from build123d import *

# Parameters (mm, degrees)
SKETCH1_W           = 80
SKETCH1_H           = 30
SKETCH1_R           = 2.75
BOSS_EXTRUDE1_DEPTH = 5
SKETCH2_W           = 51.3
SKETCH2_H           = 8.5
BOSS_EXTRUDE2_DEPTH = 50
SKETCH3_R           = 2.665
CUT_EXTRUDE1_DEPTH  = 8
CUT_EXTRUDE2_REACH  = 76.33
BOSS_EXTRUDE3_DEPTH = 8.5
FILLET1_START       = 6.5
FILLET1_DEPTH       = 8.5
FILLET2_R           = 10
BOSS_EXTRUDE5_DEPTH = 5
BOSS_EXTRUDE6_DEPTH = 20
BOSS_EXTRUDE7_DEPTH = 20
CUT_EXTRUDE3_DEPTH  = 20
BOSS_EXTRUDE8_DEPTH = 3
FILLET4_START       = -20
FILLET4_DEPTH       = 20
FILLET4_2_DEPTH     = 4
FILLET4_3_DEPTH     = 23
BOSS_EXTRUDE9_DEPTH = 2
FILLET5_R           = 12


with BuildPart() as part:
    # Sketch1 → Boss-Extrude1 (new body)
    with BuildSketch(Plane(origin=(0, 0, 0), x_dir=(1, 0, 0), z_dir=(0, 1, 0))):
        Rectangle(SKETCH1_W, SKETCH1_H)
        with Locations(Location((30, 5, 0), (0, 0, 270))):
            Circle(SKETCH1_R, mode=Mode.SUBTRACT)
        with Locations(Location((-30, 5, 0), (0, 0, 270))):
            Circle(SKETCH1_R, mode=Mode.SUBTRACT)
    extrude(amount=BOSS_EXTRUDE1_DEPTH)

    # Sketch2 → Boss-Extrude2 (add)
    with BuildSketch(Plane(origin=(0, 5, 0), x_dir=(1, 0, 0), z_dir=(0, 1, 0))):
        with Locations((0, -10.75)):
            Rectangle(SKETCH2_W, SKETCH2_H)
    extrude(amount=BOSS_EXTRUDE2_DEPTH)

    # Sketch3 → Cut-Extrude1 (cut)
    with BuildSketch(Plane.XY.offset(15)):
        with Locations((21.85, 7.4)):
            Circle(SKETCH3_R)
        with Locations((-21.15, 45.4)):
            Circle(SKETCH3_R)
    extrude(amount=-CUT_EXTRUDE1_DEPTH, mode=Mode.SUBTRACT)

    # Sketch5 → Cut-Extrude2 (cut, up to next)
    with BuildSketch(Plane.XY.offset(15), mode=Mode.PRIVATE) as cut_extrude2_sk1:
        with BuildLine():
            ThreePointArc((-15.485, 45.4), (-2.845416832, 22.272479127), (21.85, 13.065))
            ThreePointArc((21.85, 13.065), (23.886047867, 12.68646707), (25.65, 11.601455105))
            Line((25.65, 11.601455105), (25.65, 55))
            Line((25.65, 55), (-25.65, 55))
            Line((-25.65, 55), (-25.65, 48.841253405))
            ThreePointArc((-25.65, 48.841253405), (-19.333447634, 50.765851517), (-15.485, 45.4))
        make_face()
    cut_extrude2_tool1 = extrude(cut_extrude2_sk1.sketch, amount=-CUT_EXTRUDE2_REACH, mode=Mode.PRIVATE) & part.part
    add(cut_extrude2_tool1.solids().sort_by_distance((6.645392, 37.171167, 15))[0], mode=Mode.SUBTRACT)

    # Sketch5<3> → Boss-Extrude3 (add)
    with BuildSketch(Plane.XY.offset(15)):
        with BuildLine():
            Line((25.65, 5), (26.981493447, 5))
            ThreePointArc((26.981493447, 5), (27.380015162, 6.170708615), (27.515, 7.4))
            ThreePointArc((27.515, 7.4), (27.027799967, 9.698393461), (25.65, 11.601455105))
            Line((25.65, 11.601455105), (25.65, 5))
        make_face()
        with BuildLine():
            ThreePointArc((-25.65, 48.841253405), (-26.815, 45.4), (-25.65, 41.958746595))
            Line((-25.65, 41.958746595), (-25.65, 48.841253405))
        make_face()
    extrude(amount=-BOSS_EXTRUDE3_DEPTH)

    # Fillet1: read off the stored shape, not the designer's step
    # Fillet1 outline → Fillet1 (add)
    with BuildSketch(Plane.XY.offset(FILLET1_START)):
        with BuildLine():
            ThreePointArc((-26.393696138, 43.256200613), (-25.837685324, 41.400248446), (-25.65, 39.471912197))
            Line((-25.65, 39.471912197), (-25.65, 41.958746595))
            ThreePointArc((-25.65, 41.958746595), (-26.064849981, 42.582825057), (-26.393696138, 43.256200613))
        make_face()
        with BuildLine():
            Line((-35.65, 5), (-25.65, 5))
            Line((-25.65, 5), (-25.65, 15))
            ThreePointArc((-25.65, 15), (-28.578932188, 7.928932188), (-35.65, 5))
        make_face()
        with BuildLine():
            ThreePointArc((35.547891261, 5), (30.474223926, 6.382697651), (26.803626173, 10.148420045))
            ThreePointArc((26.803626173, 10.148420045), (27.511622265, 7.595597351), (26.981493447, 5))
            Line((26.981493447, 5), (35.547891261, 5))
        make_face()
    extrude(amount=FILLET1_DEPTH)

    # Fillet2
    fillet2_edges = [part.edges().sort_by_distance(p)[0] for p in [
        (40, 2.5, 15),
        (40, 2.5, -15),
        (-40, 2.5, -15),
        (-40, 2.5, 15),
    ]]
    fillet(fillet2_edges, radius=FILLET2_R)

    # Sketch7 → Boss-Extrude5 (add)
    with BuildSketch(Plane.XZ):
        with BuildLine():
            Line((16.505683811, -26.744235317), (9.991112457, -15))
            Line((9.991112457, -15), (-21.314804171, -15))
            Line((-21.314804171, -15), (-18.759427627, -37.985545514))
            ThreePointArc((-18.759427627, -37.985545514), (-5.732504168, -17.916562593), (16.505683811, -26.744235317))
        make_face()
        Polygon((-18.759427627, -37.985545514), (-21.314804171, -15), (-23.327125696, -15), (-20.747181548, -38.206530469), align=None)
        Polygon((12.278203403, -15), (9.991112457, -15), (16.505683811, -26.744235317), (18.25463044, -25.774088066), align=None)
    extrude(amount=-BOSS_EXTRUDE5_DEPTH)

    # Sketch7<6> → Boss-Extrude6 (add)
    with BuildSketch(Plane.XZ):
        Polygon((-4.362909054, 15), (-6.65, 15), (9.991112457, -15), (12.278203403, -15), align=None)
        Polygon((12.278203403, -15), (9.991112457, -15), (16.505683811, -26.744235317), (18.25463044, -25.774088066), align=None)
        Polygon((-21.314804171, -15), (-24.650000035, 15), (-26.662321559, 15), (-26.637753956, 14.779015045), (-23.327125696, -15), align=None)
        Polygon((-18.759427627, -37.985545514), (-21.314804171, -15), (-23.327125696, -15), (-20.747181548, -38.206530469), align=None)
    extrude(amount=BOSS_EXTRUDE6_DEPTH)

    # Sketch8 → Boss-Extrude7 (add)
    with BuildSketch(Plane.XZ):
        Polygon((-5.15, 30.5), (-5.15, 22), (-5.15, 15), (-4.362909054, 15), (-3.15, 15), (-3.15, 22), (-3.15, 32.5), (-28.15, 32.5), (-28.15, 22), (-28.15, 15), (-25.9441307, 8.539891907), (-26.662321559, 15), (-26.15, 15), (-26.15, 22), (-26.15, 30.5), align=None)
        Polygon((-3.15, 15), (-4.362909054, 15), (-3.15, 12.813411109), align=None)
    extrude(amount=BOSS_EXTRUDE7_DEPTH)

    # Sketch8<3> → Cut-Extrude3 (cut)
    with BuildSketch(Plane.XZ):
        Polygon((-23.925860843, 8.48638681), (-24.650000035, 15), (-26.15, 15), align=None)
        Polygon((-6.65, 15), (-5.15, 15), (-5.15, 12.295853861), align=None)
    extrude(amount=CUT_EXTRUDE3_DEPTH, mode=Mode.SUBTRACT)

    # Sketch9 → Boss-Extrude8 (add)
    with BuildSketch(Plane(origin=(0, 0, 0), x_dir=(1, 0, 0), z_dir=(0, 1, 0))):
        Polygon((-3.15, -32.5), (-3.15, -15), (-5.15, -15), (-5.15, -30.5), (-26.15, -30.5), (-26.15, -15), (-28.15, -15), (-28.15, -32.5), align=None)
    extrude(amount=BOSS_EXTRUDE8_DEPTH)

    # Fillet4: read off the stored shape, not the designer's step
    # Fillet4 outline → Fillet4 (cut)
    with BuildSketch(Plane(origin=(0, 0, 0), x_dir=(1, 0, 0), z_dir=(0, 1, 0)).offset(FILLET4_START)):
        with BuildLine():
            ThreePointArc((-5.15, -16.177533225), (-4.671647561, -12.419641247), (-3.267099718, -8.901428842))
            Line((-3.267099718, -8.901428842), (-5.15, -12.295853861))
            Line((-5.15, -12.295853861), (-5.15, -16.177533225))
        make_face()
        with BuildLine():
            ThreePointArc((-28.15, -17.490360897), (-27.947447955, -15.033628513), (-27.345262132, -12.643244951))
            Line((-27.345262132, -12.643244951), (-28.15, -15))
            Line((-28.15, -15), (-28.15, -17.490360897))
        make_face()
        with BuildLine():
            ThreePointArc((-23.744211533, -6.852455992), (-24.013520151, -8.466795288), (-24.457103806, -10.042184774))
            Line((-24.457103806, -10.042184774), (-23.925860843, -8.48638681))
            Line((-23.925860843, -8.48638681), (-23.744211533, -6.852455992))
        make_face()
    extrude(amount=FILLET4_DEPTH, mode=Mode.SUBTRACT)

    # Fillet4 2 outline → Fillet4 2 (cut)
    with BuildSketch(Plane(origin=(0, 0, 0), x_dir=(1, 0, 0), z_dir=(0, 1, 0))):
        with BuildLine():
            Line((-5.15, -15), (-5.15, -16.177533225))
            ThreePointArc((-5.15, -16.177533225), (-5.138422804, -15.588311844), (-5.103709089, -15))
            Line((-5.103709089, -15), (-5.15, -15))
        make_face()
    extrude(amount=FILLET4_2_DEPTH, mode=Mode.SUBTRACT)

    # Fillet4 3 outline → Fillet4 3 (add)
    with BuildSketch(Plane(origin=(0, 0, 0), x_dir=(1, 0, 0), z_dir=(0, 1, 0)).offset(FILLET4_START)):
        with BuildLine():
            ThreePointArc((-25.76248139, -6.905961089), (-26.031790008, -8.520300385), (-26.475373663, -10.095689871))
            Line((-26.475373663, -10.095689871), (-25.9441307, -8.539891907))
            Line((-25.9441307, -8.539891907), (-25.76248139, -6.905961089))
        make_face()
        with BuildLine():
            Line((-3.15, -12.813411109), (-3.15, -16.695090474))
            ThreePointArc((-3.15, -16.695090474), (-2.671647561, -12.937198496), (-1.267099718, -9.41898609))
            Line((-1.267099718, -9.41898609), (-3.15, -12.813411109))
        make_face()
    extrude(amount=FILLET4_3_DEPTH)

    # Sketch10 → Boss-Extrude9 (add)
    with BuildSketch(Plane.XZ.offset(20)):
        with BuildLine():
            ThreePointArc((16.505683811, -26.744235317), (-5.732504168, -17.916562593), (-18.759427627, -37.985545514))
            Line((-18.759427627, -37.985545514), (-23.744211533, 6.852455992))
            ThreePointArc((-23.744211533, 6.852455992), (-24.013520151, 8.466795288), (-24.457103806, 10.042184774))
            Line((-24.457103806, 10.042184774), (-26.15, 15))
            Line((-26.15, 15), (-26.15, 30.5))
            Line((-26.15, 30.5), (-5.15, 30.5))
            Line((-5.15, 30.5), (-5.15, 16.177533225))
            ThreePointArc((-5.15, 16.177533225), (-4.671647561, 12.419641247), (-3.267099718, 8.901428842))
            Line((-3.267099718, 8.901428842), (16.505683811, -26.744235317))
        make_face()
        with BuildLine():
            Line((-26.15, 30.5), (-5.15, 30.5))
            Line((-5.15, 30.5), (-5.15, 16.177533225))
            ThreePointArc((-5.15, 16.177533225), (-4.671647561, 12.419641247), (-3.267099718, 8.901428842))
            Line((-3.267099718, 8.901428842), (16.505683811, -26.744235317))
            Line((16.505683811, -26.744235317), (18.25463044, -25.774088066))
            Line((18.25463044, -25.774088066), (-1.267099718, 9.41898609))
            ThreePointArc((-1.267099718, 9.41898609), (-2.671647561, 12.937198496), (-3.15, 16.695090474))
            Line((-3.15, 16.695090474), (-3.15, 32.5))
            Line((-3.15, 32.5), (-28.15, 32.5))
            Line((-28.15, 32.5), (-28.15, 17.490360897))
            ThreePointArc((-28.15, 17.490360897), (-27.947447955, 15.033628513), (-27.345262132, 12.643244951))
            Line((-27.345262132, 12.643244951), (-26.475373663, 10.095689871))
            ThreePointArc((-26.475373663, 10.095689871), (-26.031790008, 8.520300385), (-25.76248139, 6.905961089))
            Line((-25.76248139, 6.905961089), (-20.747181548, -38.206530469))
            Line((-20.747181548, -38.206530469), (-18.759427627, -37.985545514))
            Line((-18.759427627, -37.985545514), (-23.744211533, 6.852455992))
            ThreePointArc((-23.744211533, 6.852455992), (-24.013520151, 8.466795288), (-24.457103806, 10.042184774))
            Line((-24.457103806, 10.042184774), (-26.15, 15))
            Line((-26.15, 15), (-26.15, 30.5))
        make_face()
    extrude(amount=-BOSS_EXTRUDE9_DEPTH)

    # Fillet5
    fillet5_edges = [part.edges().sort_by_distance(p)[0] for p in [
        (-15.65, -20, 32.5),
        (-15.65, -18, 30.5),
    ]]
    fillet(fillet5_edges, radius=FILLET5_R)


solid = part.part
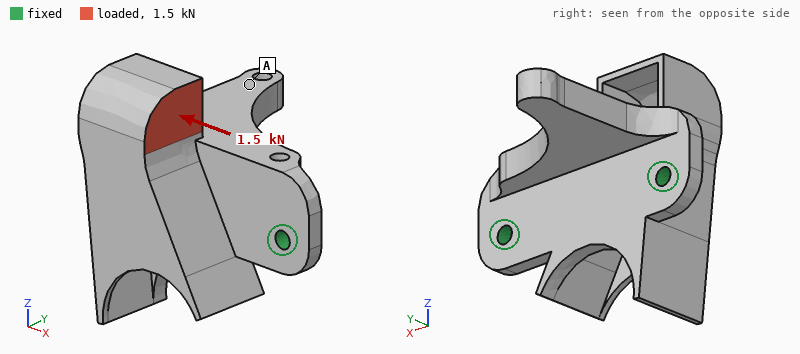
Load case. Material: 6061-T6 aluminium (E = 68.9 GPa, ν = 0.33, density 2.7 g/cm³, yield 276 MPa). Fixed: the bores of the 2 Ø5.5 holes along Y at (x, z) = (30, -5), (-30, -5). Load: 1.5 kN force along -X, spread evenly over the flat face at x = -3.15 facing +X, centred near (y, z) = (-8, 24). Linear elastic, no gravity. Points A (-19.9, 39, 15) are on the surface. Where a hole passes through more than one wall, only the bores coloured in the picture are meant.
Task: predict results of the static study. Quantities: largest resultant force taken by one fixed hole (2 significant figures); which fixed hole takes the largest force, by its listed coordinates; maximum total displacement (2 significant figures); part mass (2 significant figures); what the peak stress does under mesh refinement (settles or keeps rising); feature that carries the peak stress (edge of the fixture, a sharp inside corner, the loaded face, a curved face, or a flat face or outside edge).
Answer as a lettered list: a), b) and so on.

a) 1.2 kN
b) (30, -5)
c) 0.23 mm
d) 83 g
e) keeps rising
f) a sharp inside corner
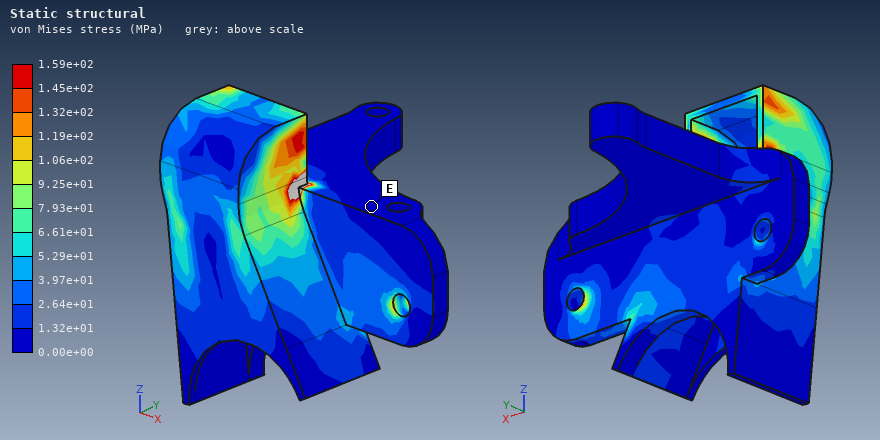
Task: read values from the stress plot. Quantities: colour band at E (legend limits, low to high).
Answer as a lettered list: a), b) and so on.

a) 0.00e+00 to 1.32e+01 MPa
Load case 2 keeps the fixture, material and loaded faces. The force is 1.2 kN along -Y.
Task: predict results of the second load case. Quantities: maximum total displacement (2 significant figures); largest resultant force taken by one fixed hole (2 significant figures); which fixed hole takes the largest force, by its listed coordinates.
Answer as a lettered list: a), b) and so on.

a) 0.28 mm
b) 660 N
c) (-30, -5)
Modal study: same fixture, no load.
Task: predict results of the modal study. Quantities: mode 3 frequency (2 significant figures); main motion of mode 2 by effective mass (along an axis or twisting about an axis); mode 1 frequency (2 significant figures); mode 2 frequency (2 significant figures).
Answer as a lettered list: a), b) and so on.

a) 4600 Hz
b) along X
c) 2000 Hz
d) 3400 Hz
